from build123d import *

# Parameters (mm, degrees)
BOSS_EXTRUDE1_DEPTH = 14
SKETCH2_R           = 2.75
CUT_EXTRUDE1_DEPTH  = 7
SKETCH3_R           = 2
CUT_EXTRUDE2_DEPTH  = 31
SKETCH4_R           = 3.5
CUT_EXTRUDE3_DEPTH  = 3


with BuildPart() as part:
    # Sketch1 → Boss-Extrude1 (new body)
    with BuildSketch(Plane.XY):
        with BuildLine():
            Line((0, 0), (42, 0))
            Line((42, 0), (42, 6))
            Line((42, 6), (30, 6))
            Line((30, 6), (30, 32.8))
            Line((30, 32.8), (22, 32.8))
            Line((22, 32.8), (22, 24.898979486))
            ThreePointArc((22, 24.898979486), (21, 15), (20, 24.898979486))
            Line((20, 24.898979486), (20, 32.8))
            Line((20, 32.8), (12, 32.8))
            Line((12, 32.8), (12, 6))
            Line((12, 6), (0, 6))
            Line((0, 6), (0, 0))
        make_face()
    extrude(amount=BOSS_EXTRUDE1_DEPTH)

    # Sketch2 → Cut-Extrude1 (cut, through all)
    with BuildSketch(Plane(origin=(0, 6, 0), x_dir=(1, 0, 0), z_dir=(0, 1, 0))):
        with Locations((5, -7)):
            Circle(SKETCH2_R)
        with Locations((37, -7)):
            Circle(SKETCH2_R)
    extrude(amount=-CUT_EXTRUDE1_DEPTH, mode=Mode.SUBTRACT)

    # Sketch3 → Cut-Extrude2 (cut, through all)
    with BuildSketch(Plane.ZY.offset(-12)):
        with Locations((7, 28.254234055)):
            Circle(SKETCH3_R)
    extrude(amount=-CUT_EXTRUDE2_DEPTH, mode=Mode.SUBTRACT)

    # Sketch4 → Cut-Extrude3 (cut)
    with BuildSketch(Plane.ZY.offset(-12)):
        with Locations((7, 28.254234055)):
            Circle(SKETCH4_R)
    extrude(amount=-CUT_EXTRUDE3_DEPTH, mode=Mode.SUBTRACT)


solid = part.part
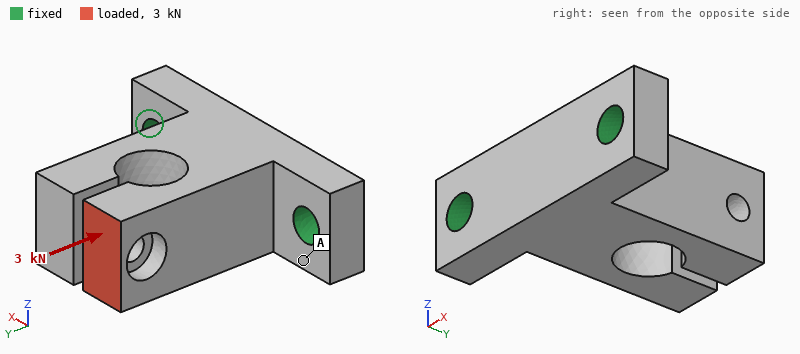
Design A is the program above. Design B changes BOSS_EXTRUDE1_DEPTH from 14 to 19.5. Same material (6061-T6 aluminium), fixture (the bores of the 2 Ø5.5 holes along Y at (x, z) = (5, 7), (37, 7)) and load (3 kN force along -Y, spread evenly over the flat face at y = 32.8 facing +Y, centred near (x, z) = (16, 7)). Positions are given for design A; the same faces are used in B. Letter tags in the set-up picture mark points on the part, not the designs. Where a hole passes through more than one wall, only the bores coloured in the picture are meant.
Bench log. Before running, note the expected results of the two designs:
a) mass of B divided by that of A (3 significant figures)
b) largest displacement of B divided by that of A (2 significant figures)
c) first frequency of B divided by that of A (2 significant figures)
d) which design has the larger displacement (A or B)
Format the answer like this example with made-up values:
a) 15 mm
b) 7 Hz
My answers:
a) 1.42
b) 0.78
c) 0.98
d) A
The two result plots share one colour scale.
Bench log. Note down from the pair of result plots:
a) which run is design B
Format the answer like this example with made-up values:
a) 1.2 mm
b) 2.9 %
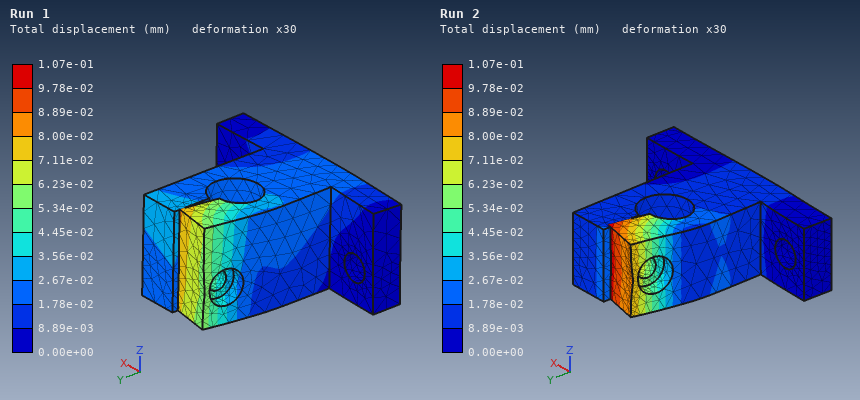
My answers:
a) Run 1
